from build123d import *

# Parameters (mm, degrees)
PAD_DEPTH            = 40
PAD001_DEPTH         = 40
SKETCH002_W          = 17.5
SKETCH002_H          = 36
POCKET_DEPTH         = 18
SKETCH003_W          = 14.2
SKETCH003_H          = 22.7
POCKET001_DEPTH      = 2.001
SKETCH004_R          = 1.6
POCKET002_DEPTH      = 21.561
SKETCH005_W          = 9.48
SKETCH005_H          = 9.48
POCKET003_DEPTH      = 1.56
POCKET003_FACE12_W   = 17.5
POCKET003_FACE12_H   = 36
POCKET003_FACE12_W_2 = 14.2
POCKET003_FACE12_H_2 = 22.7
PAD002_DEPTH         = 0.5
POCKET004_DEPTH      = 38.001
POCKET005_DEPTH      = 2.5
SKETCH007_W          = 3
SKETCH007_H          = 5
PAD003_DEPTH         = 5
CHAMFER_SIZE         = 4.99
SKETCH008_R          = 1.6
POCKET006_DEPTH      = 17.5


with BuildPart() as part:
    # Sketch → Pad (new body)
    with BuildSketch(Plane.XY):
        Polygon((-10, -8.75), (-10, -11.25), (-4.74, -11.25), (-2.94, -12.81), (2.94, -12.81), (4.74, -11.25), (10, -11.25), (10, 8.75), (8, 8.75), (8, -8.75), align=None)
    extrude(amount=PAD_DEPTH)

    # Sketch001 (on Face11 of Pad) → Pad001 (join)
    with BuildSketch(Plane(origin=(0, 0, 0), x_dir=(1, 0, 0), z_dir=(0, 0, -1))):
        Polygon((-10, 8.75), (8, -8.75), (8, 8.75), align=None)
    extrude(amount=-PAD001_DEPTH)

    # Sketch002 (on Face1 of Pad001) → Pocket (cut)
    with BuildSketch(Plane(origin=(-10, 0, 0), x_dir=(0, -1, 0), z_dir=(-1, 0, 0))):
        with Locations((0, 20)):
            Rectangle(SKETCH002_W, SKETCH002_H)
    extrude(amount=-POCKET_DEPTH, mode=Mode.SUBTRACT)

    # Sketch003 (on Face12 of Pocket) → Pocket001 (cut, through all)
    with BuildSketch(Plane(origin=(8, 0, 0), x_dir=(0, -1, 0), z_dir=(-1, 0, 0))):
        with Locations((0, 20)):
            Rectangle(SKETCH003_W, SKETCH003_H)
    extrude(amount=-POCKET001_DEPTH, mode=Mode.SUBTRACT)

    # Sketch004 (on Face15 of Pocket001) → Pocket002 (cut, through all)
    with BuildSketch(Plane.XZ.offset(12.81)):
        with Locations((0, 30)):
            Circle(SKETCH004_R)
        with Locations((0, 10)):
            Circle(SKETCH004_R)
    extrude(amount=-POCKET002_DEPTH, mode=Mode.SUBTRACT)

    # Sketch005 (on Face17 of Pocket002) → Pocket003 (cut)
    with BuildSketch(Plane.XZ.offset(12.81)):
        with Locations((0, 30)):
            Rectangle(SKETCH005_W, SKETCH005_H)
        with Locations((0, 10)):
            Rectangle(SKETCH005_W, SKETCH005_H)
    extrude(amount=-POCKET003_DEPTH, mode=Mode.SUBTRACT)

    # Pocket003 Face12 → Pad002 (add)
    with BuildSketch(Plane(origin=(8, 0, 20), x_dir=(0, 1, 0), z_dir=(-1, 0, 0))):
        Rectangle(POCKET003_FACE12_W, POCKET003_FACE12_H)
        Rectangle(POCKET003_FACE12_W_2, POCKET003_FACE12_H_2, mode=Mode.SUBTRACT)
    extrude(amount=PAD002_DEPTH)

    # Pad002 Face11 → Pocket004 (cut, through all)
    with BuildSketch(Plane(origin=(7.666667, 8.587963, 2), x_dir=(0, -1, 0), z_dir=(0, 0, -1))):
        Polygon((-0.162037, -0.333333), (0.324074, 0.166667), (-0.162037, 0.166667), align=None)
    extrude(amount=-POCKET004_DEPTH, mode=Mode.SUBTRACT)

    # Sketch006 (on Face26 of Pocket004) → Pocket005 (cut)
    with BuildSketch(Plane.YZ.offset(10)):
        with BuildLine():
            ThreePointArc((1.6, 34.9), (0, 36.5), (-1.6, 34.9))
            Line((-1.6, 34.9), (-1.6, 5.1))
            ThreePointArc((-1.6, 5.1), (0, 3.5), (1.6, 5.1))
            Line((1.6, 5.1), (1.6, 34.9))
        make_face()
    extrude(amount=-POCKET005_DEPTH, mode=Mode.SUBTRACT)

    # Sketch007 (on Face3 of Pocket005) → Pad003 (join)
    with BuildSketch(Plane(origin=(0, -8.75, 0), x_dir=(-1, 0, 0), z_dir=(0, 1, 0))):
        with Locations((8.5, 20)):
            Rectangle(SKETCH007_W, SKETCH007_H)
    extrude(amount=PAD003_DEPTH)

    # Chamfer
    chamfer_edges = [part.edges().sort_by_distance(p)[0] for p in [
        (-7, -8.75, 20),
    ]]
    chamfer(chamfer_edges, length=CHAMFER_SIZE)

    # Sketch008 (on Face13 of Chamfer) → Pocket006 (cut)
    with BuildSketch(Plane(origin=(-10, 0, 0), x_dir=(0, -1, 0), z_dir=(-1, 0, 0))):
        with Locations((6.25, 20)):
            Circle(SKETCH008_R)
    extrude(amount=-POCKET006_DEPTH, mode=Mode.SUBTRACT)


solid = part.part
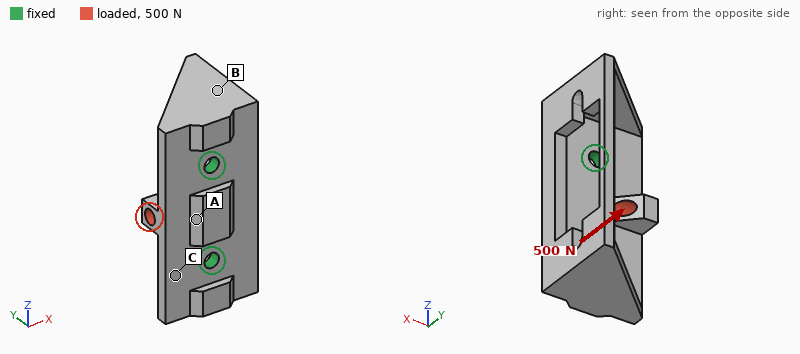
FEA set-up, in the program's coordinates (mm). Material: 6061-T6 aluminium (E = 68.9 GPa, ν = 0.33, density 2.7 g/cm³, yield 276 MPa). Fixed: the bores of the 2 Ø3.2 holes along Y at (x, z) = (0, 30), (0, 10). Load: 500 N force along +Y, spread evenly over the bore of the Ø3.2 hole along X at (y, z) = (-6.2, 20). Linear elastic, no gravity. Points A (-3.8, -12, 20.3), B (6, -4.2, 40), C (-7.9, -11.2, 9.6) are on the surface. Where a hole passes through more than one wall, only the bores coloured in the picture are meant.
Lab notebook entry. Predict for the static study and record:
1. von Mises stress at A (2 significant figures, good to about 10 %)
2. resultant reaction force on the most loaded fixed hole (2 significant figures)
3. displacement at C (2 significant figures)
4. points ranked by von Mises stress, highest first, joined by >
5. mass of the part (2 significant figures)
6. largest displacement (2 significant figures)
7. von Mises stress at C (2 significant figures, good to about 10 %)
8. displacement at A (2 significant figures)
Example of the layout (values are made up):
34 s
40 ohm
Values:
57 MPa
260 N
18 µm
A > C > B
10 g
66 µm
44 MPa
24 µm
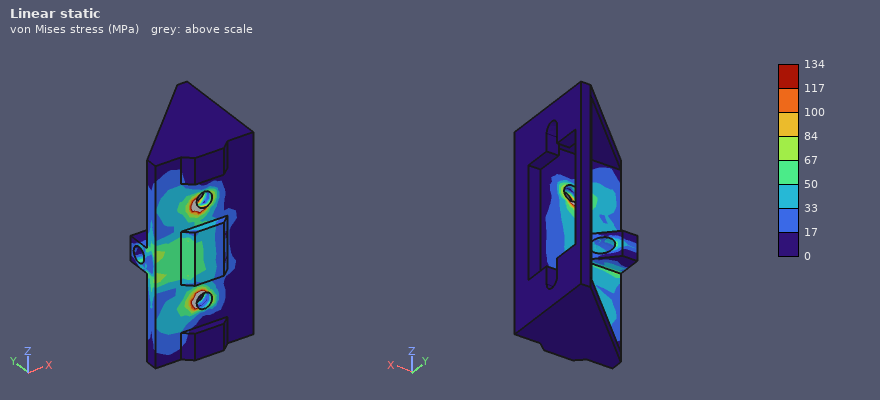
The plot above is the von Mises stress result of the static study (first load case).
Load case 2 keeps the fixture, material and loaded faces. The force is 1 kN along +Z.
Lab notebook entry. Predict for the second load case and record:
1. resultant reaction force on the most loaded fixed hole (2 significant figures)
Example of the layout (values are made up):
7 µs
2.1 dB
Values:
630 N
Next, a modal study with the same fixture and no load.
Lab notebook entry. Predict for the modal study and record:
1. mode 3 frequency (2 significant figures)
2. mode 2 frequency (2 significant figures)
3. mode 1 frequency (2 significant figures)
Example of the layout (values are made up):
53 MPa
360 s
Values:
8200 Hz
5500 Hz
5300 Hz
